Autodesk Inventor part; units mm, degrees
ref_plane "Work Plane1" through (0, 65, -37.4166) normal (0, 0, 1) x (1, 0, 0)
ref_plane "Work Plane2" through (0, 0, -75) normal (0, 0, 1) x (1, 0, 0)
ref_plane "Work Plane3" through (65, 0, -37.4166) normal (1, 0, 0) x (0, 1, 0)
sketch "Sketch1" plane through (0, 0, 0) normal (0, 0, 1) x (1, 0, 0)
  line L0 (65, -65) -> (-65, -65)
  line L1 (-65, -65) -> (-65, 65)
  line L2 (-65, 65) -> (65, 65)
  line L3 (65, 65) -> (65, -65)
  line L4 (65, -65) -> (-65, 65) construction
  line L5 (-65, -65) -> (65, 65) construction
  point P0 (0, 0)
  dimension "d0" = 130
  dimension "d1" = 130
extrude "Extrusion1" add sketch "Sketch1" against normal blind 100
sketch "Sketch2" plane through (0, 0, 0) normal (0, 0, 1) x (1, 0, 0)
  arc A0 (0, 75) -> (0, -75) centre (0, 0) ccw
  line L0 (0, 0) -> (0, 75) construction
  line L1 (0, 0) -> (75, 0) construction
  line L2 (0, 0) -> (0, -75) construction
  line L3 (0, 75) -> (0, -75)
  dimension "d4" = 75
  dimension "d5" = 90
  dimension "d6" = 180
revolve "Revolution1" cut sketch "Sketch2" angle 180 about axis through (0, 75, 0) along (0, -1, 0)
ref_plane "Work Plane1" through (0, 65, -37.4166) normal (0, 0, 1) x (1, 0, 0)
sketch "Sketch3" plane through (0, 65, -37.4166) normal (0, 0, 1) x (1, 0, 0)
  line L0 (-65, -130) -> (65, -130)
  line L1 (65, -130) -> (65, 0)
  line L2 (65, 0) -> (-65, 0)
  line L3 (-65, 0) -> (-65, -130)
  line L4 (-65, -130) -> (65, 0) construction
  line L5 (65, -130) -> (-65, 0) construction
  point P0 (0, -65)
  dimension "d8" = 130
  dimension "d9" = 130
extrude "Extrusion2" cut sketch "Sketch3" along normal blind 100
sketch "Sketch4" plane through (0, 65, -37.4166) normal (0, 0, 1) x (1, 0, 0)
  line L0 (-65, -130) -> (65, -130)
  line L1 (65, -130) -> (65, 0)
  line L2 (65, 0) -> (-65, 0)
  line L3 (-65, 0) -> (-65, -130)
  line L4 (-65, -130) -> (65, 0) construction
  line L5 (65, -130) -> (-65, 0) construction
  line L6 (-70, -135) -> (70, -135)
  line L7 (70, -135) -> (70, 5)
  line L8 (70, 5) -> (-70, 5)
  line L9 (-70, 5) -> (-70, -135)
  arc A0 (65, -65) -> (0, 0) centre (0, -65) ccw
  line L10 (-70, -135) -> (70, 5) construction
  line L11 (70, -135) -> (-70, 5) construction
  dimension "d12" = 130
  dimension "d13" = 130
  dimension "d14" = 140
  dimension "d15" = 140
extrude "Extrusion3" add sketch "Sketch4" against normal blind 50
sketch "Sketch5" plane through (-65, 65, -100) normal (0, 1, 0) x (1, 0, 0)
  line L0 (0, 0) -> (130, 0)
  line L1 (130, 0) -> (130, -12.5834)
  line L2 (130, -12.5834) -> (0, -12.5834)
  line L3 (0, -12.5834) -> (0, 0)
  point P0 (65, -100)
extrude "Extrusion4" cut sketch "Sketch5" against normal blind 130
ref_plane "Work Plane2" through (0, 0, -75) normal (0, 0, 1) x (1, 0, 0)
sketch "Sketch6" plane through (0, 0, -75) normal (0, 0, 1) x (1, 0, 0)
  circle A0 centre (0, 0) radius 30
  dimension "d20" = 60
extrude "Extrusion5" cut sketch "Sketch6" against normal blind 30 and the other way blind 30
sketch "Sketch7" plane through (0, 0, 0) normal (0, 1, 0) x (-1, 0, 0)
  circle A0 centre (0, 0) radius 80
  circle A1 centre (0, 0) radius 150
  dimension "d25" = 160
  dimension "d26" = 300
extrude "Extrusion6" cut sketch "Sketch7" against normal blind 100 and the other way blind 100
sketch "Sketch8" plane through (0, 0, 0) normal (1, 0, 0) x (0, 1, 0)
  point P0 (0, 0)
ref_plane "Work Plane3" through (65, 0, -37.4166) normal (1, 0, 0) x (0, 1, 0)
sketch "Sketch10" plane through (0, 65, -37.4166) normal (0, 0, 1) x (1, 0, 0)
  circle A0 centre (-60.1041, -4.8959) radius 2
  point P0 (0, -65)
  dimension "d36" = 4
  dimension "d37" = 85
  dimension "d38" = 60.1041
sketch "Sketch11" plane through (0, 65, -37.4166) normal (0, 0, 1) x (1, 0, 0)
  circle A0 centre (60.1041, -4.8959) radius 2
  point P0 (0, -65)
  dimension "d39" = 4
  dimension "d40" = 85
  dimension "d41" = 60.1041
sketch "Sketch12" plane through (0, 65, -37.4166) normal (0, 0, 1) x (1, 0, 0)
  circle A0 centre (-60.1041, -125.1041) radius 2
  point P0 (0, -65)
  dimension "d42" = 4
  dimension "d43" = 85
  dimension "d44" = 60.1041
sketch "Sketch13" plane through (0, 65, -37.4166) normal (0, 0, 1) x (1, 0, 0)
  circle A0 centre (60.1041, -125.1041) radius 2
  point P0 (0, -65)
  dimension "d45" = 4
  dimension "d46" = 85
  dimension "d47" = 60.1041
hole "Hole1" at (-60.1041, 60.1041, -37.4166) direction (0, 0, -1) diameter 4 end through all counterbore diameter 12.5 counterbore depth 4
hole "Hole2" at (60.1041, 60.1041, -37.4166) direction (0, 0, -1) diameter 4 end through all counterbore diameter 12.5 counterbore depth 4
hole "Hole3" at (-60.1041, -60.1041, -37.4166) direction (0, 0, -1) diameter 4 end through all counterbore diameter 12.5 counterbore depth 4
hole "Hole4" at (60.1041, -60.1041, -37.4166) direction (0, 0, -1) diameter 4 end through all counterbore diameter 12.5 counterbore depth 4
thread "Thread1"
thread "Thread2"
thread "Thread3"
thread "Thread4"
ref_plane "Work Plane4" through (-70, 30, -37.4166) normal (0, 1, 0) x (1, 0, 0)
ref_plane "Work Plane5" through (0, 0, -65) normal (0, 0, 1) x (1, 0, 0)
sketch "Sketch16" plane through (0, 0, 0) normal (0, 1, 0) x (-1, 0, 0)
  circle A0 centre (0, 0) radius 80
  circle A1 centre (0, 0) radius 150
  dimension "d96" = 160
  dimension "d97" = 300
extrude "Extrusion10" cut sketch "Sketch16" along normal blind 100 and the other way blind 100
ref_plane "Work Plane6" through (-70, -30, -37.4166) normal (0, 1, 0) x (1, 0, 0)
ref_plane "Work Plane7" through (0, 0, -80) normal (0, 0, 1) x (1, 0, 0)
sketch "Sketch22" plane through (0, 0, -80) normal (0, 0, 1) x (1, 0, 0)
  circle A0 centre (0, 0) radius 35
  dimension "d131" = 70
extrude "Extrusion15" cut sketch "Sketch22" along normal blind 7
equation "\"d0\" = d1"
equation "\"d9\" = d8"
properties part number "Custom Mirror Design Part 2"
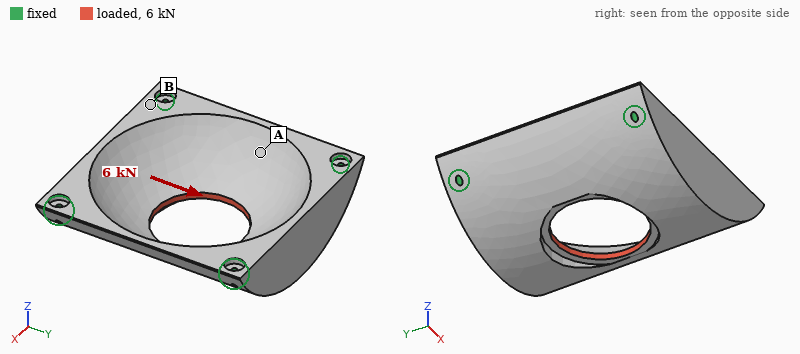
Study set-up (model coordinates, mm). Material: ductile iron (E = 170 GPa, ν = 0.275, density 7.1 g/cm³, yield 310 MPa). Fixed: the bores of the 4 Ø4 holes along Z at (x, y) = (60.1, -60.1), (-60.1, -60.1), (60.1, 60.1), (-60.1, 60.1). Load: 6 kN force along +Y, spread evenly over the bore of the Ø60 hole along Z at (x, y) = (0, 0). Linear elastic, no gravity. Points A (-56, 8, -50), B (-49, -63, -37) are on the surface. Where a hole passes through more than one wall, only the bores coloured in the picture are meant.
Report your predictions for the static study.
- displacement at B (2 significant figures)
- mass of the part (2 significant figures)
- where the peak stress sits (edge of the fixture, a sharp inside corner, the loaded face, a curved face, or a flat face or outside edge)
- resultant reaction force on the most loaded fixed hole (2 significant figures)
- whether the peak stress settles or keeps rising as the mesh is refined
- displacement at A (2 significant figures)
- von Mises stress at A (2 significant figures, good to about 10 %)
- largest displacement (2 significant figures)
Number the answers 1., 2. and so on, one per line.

1. 0.88 µm
2. 2.1 kg
3. edge of the fixture
4. 1.7 kN
5. keeps rising
6. 1.2 µm
7. 6.2 MPa
8. 3.9 µm
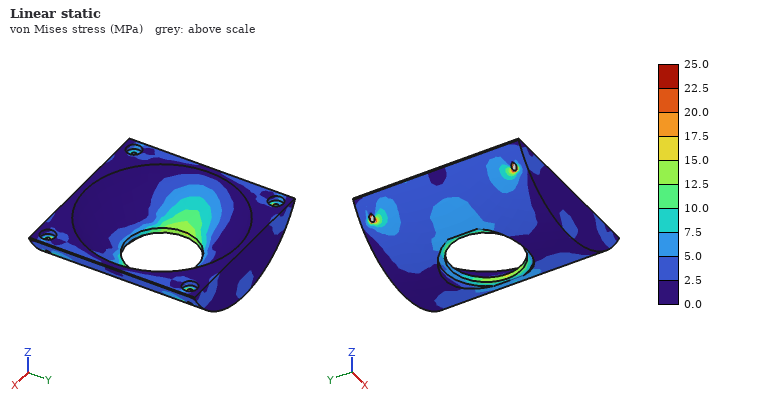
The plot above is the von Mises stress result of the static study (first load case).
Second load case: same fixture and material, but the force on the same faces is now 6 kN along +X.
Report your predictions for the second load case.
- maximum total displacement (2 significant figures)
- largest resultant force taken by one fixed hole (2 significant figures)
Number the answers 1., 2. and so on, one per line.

1. 10 µm
2. 1.7 kN
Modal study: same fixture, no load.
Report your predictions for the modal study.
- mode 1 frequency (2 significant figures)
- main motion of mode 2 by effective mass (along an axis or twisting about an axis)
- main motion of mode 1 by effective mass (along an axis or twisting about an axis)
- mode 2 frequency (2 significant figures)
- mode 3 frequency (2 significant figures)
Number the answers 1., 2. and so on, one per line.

1. 4200 Hz
2. along Z
3. along Z
4. 4800 Hz
5. 5300 Hz
